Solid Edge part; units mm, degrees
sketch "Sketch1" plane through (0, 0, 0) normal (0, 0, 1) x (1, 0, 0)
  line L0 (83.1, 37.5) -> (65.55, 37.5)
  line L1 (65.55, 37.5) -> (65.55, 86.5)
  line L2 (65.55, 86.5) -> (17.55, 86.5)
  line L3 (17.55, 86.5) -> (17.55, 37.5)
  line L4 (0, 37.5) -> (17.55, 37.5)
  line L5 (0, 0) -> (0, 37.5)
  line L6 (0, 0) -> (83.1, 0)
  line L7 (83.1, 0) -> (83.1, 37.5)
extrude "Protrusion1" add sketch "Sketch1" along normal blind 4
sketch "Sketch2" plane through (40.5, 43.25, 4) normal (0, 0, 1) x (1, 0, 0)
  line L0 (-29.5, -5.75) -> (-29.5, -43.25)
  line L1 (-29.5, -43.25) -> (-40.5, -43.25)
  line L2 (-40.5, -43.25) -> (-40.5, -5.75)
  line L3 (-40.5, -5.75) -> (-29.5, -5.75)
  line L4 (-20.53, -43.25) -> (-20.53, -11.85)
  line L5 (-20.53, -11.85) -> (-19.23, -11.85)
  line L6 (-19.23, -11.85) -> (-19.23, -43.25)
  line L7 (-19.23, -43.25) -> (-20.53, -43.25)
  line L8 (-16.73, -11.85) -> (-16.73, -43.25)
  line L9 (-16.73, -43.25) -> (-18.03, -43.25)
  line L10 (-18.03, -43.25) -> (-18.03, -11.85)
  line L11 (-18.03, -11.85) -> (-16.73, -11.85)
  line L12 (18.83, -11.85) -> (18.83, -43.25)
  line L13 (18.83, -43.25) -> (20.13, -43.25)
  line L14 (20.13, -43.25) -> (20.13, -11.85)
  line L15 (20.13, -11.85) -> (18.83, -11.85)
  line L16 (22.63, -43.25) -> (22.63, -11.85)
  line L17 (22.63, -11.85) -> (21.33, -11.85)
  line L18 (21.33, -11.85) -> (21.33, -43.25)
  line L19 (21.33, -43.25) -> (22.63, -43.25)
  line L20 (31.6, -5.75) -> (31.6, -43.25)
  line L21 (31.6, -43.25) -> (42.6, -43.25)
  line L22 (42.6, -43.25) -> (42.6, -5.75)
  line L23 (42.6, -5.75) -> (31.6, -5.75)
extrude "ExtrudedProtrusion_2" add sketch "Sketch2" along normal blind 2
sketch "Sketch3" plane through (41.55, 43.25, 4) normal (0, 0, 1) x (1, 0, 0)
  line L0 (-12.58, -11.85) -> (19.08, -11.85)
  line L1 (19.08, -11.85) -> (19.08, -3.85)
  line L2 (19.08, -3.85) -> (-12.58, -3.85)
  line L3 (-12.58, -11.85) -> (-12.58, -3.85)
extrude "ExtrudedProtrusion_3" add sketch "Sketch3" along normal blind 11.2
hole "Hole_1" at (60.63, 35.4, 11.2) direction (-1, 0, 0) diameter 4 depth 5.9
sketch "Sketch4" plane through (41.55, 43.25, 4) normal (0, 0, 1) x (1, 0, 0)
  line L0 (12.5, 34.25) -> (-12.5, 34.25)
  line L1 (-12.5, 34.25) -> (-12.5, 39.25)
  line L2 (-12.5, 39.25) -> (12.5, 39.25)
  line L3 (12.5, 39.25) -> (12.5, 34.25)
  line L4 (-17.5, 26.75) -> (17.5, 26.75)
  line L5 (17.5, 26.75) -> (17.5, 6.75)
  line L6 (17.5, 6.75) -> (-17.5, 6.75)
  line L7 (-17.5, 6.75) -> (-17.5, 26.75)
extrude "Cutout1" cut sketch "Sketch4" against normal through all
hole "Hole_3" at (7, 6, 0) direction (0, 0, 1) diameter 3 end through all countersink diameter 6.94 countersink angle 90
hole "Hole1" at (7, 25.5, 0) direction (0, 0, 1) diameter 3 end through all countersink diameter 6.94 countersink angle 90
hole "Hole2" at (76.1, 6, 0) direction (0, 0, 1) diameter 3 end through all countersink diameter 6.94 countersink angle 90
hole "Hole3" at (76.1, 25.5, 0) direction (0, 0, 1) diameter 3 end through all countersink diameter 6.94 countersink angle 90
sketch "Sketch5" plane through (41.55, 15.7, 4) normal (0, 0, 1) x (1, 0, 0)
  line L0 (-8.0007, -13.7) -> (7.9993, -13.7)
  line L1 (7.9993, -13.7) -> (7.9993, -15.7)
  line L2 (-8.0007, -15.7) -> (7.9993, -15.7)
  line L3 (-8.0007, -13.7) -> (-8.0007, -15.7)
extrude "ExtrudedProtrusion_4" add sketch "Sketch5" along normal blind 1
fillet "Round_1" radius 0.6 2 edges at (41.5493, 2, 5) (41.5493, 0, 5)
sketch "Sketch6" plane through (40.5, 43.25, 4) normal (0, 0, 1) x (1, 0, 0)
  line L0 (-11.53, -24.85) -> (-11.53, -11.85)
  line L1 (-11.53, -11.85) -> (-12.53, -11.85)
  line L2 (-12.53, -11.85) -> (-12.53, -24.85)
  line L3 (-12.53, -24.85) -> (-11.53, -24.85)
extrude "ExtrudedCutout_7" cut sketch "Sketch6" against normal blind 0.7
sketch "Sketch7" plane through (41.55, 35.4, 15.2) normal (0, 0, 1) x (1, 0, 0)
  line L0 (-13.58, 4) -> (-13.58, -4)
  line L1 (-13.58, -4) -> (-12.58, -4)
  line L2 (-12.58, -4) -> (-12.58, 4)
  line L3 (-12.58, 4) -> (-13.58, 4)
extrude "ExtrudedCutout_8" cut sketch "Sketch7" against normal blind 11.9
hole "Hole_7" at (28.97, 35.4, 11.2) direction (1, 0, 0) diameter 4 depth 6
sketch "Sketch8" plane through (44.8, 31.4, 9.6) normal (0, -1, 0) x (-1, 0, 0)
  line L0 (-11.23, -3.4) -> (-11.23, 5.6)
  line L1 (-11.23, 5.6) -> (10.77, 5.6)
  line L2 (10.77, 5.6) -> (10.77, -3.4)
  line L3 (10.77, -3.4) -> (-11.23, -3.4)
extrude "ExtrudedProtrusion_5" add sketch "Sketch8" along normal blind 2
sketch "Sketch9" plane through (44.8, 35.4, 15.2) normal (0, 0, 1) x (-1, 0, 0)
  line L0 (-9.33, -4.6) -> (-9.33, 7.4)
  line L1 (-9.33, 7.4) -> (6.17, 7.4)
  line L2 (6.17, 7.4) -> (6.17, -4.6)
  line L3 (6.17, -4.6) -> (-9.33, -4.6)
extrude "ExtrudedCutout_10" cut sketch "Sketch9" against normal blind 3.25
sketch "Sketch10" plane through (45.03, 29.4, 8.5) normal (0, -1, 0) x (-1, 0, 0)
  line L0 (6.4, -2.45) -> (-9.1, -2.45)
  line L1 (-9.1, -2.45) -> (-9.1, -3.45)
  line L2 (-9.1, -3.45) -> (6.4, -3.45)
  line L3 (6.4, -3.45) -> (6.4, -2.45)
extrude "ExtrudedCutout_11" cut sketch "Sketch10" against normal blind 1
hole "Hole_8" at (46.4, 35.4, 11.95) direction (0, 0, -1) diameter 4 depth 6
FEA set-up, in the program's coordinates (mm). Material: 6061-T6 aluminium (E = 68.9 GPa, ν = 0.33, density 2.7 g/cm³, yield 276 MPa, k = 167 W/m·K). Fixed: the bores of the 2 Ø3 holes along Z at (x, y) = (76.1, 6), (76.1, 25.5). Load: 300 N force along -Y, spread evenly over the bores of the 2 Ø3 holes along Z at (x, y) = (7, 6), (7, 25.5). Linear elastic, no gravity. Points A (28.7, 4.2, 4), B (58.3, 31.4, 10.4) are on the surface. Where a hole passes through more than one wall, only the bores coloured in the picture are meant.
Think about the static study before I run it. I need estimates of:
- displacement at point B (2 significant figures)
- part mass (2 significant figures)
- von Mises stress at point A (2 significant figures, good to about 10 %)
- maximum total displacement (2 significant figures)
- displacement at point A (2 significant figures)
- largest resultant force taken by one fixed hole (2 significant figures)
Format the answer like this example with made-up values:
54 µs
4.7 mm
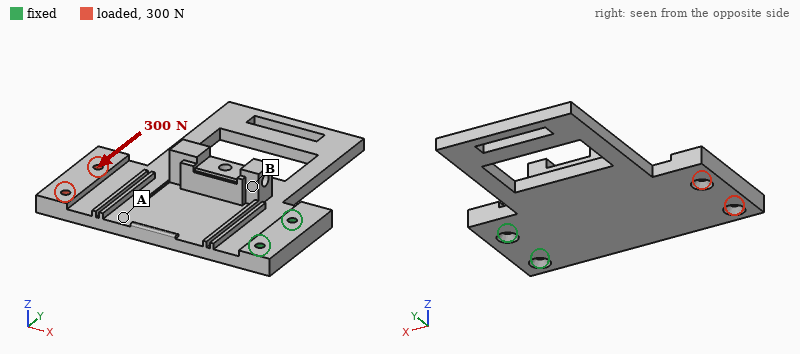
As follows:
17 µm
62 g
6.9 MPa
91 µm
32 µm
990 N
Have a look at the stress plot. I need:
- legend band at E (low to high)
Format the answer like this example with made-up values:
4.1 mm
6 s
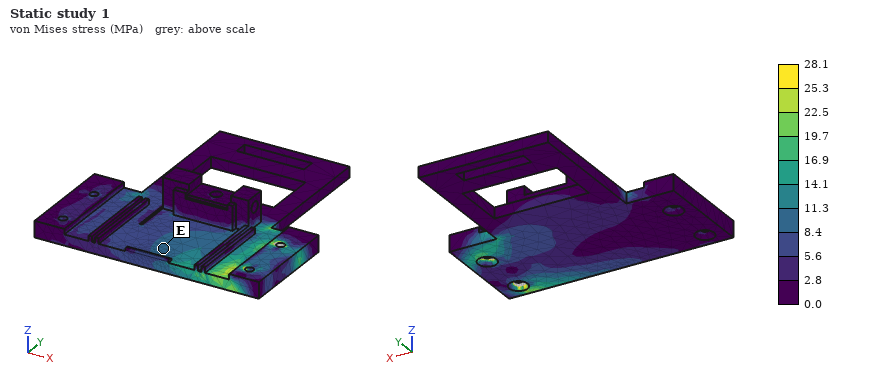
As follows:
8.4 to 11.3 MPa
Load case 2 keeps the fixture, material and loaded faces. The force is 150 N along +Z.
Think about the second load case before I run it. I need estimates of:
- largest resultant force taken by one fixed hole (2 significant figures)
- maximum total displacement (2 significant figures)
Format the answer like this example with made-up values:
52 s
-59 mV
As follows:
120 N
1.0 mm
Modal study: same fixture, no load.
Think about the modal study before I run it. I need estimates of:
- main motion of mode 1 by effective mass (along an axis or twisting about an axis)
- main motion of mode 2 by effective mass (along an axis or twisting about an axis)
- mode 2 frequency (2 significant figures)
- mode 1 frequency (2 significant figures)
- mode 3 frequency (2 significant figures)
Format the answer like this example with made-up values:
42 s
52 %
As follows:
along Z
twisting about X
770 Hz
470 Hz
2100 Hz
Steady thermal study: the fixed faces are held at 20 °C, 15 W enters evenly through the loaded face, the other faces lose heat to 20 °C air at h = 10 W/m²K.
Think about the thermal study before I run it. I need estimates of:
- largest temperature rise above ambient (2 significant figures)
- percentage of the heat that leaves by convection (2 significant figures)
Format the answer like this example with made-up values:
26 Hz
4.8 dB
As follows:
36 K
14 %
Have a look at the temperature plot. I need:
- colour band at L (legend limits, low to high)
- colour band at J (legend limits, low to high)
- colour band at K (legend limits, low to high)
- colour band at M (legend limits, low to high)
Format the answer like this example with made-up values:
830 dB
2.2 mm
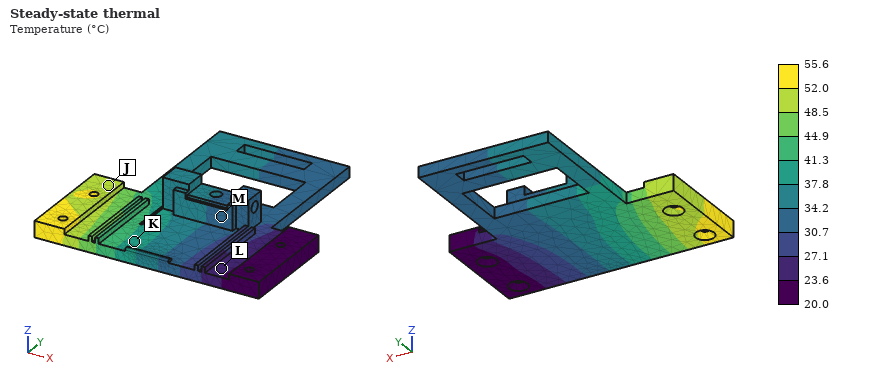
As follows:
23.6 to 27.1 °C
48.5 to 52.0 °C
37.8 to 41.3 °C
30.7 to 34.2 °C
